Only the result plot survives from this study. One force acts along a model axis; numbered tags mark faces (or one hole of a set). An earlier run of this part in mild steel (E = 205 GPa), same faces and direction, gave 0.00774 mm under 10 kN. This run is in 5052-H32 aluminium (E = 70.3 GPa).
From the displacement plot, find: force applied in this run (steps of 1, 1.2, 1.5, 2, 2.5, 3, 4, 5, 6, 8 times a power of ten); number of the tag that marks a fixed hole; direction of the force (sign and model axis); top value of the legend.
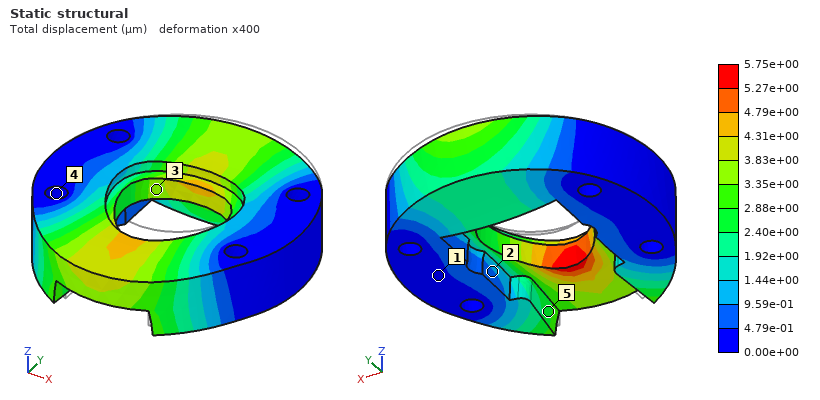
2.5 kN
4
-Y
5.75e+00 µm
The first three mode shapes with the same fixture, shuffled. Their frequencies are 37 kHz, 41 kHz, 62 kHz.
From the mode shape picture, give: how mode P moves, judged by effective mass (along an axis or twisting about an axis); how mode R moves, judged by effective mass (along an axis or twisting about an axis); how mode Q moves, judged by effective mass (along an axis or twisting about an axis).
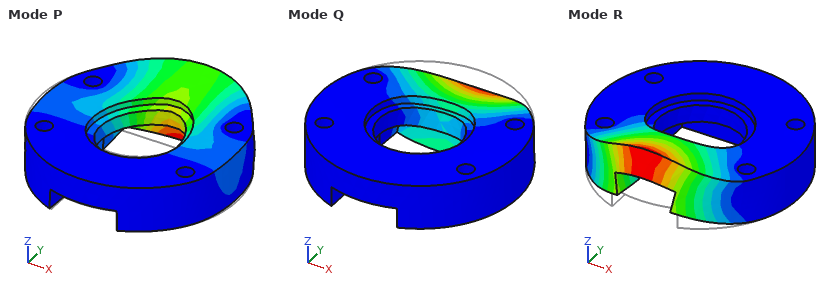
along Y
along Z
along Z
